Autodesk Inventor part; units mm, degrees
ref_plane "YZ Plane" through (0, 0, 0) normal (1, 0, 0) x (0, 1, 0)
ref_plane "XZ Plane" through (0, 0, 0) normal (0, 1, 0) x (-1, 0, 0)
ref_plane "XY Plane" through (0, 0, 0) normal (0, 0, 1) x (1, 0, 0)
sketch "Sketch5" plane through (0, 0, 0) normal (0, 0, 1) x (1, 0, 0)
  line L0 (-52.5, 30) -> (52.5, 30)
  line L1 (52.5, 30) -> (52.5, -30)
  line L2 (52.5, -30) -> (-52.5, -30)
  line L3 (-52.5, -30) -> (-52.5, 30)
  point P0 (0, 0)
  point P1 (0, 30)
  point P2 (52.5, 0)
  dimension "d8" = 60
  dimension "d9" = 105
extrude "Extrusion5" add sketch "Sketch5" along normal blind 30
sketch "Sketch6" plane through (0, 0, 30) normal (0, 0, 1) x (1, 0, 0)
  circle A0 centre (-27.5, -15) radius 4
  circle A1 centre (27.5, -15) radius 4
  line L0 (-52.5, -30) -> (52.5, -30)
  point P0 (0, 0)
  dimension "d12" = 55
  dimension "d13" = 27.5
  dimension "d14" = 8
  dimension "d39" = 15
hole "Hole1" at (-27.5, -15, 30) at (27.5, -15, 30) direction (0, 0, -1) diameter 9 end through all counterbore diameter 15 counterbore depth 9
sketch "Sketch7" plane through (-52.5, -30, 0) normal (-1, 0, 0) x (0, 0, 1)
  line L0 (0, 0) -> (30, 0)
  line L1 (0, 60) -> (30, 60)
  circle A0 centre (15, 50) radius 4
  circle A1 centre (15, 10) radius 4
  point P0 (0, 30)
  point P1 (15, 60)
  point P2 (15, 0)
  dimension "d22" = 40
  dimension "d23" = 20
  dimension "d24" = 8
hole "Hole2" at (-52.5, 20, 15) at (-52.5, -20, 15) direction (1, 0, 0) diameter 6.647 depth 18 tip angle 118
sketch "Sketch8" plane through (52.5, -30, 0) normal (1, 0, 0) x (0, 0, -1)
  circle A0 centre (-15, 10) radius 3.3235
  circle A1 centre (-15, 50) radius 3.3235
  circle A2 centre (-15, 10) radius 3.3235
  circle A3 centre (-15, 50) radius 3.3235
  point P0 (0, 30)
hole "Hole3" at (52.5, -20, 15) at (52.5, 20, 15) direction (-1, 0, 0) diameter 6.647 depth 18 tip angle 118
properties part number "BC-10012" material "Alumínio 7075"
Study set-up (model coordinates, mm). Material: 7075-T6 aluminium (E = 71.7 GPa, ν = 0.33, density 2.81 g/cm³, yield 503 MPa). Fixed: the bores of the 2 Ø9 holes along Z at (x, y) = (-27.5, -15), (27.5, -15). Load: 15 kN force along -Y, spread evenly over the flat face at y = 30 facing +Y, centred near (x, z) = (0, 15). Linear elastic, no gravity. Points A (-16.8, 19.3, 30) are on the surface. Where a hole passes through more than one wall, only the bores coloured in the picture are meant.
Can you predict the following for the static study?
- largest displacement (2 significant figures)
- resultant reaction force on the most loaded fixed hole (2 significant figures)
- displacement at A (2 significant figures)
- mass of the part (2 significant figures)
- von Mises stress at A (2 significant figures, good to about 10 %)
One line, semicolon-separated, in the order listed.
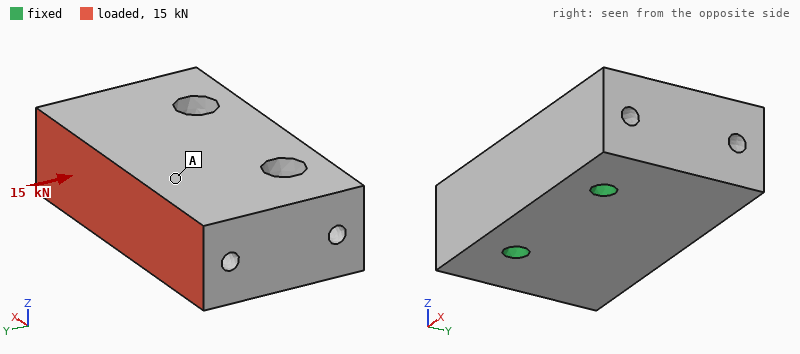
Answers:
10.0 µm; 7.5 kN; 8.0 µm; 510 g; 5.0 MPa
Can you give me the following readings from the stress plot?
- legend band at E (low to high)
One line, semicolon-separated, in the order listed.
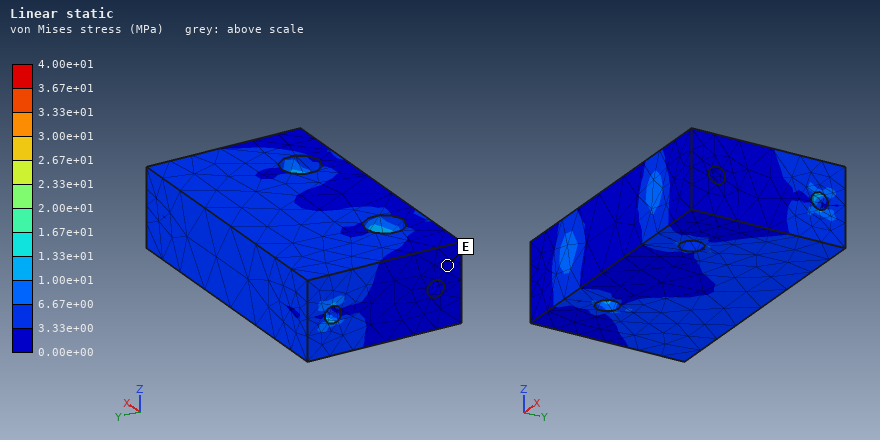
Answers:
0.00e+00 to 3.33e+00 MPa
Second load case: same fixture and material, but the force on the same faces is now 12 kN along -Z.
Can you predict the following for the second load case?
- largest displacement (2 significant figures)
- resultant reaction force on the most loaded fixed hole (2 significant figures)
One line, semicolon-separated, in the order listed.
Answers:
75 µm; 6.0 kN
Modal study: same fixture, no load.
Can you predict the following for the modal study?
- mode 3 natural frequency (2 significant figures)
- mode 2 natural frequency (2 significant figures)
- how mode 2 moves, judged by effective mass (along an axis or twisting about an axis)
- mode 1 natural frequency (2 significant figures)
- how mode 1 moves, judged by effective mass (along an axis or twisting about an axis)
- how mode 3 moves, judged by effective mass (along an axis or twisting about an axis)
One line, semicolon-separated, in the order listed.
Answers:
10 kHz; 8700 Hz; twisting about Y; 5700 Hz; along Z; along X
